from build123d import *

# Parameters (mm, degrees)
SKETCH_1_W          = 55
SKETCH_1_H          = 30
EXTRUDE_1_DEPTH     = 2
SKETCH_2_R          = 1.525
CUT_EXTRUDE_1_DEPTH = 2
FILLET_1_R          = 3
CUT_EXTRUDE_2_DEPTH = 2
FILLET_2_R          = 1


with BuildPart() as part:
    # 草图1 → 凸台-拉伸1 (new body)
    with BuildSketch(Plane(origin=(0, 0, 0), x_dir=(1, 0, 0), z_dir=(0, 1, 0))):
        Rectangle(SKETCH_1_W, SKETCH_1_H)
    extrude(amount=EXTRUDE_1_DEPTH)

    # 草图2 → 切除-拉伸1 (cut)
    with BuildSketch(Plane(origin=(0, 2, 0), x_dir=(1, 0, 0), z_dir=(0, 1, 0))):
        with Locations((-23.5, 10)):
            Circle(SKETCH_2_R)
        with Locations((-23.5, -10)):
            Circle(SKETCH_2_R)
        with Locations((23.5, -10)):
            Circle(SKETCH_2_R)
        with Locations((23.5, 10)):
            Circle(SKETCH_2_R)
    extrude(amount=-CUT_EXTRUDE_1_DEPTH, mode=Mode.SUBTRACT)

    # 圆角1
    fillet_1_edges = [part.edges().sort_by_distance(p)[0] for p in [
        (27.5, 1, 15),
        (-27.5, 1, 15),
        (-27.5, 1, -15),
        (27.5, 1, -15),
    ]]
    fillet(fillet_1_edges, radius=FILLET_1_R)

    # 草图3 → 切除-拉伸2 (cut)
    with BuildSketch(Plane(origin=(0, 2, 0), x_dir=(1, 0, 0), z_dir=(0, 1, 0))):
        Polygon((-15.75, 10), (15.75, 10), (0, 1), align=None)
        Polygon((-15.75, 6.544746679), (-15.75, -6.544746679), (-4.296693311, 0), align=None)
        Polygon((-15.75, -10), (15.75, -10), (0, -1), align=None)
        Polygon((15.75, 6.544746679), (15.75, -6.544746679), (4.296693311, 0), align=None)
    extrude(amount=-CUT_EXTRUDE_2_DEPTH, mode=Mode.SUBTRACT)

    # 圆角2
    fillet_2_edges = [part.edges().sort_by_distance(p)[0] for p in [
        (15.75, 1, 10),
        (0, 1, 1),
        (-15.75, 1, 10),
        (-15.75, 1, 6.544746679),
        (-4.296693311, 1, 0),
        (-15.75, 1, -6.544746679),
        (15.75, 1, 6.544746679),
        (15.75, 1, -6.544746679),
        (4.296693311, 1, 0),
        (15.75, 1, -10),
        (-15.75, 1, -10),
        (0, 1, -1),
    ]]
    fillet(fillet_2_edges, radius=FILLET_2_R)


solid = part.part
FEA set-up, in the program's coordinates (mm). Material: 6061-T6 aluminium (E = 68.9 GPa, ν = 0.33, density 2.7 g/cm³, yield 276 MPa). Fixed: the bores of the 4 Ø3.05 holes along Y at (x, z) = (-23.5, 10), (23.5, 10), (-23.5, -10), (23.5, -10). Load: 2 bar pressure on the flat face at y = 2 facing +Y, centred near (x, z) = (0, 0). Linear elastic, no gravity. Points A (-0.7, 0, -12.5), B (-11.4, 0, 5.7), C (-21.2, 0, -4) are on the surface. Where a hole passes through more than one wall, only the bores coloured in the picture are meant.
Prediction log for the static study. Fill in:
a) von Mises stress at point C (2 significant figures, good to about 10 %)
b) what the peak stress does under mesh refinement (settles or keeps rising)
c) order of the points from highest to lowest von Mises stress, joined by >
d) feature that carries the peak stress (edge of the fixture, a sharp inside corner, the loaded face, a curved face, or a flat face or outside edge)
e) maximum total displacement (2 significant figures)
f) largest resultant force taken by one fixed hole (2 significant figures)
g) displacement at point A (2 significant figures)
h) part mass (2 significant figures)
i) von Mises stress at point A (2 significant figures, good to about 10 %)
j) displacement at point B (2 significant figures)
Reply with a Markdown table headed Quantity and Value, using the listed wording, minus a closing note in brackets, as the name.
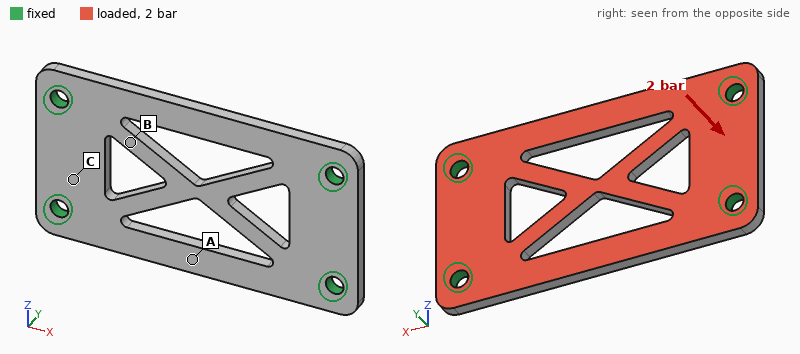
| Quantity | Value |
|---|---|
| von Mises stress at point C | 13 MPa |
| what the peak stress does under mesh refinement | keeps rising |
| order of the points from highest to lowest von Mises stress, joined by > | A > C > B |
| feature that carries the peak stress | edge of the fixture |
| maximum total displacement | 49 µm |
| largest resultant force taken by one fixed hole | 60 N |
| displacement at point A | 42 µm |
| part mass | 6.4 g |
| von Mises stress at point A | 23 MPa |
| displacement at point B | 25 µm |
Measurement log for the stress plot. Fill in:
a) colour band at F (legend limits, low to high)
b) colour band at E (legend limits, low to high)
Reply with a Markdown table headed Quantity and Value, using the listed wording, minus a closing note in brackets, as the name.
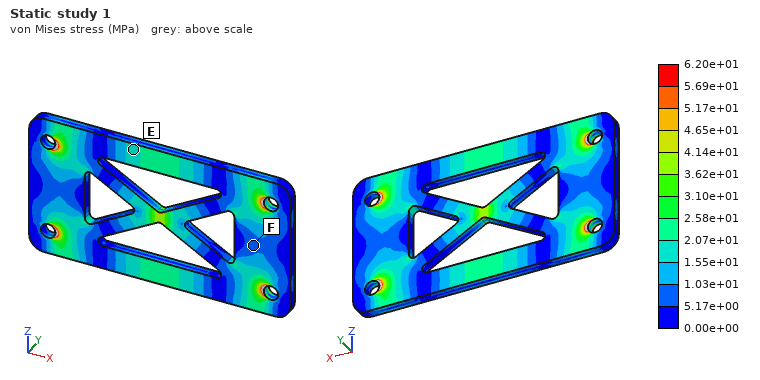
| Quantity | Value |
|---|---|
| colour band at F | 5.17e+00 to 1.03e+01 MPa |
| colour band at E | 1.55e+01 to 2.07e+01 MPa |
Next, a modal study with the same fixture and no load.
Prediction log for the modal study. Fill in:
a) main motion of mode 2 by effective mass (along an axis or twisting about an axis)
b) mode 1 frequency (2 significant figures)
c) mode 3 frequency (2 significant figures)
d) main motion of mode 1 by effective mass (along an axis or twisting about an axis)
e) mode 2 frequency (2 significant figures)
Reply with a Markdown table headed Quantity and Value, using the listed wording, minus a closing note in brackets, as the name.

| Quantity | Value |
|---|---|
| main motion of mode 2 by effective mass | twisting about X |
| mode 1 frequency | 5400 Hz |
| mode 3 frequency | 8300 Hz |
| main motion of mode 1 by effective mass | along Y |
| mode 2 frequency | 6300 Hz |
